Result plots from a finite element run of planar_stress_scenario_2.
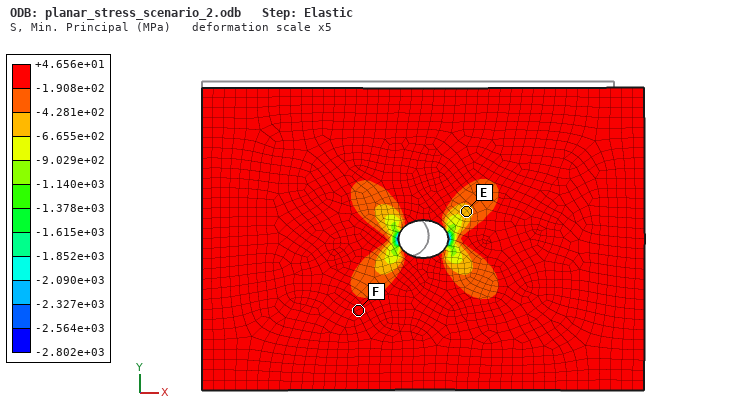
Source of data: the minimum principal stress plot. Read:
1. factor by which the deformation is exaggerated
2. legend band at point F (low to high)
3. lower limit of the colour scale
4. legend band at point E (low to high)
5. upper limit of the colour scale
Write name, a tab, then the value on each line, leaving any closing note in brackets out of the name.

factor by which the deformation is exaggerated	5
legend band at point F	-1.908e+02 to +4.656e+01 MPa
lower limit of the colour scale	-2.802e+03 MPa
legend band at point E	-6.655e+02 to -4.281e+02 MPa
upper limit of the colour scale	+4.656e+01 MPa
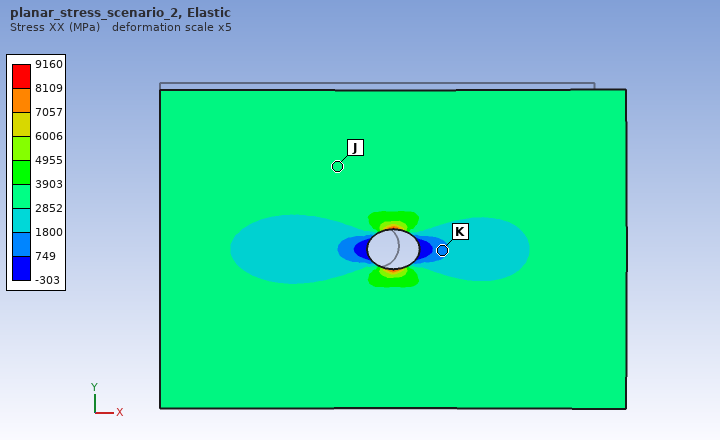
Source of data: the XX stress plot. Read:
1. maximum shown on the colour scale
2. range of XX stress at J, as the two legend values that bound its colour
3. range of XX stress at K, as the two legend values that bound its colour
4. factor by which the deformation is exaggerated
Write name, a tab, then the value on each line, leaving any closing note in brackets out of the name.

maximum shown on the colour scale	9160 MPa
range of XX stress at J, as the two legend values that bound its colour	2852 to 3903 MPa
range of XX stress at K, as the two legend values that bound its colour	749 to 1800 MPa
factor by which the deformation is exaggerated	5
